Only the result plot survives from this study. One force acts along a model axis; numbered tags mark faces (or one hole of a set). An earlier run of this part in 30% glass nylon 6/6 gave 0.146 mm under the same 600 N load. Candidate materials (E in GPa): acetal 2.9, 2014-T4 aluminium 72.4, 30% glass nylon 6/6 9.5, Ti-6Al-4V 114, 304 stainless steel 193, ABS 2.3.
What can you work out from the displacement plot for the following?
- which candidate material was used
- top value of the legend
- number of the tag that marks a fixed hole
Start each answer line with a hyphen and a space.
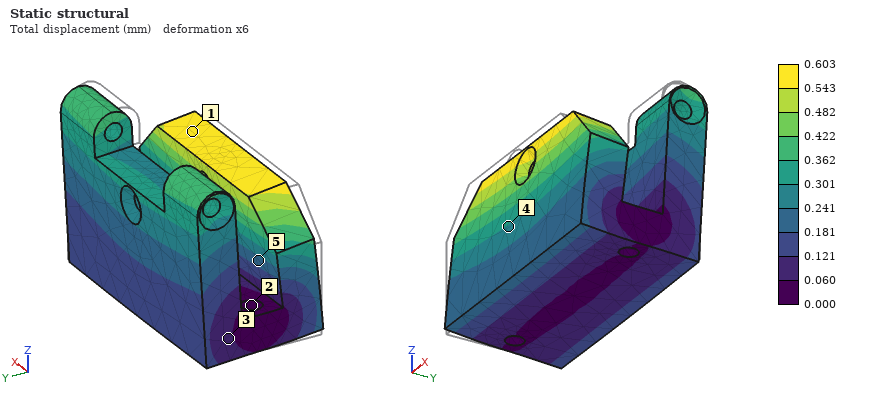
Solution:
- ABS
- 0.603 mm
- 2
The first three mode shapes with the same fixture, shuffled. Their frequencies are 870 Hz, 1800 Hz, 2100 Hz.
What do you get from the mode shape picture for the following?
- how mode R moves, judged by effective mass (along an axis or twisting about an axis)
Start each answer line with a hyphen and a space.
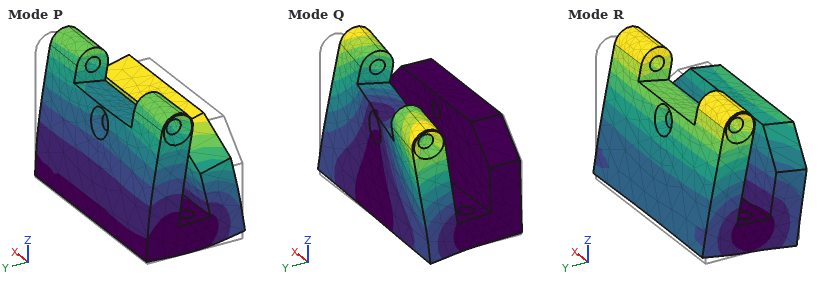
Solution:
- along Y
